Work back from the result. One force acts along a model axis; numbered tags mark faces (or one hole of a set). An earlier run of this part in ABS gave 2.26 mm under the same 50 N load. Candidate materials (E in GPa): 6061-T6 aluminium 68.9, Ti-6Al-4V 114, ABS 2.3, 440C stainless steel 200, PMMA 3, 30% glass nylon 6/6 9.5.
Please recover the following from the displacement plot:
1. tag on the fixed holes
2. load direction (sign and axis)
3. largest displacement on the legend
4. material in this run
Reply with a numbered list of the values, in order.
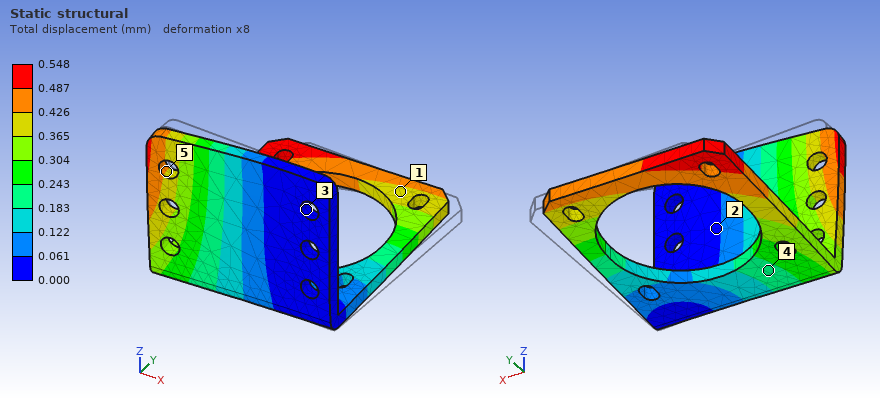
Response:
1. 3
2. -Y
3. 0.548 mm
4. 30% glass nylon 6/6
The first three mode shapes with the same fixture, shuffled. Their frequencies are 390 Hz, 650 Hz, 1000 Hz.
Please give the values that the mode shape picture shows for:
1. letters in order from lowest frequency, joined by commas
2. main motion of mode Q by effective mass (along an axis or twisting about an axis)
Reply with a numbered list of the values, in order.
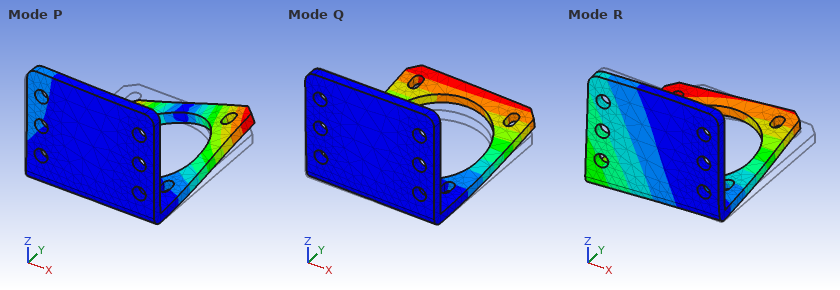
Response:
1. Q, R, P
2. along Z
